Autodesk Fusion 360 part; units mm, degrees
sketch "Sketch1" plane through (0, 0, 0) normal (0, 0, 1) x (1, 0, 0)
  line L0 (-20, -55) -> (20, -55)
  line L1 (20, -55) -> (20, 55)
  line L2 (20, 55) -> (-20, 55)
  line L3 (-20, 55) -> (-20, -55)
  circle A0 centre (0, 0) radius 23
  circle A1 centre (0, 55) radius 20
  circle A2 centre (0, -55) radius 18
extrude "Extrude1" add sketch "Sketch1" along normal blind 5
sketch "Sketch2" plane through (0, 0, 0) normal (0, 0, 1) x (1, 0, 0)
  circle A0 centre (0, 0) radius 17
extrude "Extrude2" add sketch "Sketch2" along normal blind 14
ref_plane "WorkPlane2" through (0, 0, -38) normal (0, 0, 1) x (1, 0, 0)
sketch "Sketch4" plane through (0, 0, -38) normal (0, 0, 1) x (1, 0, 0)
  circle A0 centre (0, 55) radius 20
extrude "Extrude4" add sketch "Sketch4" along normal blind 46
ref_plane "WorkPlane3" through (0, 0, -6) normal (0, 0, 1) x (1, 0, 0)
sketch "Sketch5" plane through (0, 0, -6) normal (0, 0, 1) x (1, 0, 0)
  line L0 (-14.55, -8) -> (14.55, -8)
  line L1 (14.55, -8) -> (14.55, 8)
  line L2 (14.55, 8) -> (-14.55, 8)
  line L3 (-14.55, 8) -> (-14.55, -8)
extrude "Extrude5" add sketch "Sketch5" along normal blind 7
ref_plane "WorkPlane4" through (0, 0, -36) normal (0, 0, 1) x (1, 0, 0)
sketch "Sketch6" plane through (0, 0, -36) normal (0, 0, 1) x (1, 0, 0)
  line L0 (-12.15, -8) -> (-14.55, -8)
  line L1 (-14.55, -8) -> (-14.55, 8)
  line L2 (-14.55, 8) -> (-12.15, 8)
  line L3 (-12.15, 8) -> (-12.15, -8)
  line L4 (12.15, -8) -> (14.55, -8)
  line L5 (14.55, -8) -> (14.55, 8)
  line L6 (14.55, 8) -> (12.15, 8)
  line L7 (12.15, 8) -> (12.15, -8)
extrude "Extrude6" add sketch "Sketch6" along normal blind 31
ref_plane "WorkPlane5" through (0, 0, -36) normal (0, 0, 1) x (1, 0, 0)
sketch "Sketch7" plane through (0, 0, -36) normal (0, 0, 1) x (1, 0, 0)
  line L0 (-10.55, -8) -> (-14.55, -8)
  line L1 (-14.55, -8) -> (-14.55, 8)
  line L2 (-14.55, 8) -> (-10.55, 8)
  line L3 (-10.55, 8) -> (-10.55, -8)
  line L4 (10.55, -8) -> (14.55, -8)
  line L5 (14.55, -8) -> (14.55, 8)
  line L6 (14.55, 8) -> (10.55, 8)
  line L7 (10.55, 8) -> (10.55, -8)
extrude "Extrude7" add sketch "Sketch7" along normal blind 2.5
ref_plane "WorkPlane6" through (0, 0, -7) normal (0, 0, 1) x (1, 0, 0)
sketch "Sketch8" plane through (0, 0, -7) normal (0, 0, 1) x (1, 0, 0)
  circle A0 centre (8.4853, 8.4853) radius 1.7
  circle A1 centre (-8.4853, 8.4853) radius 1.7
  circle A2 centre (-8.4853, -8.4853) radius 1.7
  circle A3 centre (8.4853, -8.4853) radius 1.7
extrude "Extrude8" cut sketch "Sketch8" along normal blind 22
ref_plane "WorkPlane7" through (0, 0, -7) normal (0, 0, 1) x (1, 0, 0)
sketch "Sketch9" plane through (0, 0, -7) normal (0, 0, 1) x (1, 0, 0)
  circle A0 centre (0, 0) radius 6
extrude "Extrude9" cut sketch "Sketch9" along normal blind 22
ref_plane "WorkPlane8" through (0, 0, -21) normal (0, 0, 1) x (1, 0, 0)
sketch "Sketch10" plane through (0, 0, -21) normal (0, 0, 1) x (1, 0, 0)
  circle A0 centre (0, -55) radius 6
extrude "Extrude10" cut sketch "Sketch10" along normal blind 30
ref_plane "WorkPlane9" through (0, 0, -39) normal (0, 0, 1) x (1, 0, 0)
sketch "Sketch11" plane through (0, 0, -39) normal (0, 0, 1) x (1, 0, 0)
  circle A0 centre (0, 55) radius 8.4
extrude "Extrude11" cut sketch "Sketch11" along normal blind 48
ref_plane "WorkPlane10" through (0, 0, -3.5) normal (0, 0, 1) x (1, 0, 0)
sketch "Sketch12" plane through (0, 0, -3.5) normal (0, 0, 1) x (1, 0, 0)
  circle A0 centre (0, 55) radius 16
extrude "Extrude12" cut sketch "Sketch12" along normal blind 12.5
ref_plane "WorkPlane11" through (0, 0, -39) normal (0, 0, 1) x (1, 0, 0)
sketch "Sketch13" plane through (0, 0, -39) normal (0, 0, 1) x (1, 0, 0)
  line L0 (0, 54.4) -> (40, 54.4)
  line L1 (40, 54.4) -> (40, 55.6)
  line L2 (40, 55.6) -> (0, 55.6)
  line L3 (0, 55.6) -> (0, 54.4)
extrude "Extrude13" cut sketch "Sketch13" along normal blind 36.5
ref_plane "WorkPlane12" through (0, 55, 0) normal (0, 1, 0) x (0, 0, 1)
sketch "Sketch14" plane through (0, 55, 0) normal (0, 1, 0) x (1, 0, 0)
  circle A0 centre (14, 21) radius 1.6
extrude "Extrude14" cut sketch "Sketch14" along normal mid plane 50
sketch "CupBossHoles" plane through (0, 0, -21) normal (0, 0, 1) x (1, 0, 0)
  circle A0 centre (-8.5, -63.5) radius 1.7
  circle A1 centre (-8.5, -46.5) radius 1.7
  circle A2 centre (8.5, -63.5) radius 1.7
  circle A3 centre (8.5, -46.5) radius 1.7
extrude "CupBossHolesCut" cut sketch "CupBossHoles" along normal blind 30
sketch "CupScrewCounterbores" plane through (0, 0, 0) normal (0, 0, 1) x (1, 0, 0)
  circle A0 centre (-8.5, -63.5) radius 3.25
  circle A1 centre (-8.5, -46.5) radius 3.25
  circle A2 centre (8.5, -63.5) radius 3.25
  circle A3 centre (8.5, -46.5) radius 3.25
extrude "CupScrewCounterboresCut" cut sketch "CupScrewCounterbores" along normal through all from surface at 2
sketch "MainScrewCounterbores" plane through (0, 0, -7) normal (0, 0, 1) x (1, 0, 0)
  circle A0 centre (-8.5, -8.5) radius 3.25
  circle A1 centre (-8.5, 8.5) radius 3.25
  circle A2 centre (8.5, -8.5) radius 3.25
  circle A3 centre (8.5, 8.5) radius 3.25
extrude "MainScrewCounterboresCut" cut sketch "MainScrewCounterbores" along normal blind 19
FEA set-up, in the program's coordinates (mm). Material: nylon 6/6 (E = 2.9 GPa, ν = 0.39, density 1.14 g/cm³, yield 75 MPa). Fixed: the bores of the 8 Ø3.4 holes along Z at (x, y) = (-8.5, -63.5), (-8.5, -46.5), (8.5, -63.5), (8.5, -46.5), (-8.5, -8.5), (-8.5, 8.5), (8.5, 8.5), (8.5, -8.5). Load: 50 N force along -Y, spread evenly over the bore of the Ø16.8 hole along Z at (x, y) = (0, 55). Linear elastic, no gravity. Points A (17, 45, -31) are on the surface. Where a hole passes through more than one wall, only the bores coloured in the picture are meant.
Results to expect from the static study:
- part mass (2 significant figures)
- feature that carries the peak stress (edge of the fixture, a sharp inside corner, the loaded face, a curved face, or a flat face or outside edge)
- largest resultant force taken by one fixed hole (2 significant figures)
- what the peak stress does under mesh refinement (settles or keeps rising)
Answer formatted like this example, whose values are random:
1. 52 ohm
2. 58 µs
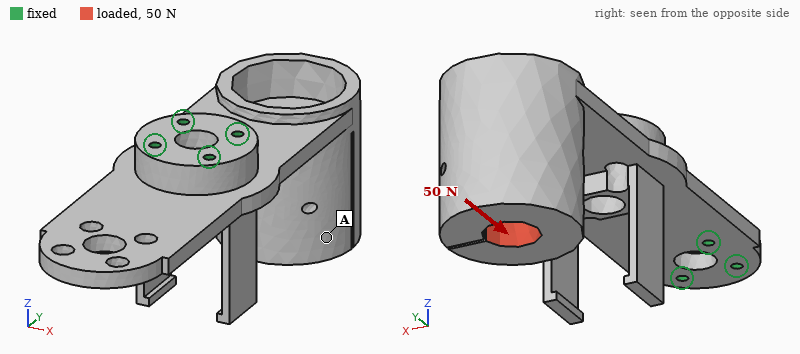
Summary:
1. 80 g
2. edge of the fixture
3. 38 N
4. keeps rising
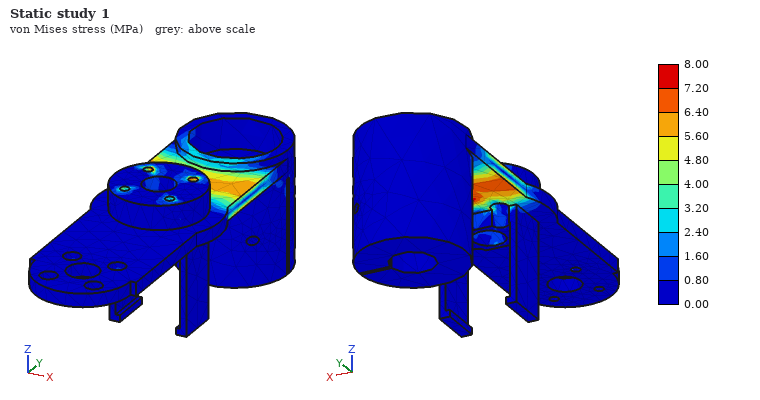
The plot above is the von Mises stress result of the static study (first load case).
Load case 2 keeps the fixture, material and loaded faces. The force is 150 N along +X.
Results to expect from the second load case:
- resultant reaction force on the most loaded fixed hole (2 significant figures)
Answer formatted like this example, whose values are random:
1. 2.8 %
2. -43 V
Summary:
1. 250 N
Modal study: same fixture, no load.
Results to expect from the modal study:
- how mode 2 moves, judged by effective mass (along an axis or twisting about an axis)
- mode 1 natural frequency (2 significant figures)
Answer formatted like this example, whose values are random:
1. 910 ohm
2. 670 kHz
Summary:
1. along X
2. 120 Hz
